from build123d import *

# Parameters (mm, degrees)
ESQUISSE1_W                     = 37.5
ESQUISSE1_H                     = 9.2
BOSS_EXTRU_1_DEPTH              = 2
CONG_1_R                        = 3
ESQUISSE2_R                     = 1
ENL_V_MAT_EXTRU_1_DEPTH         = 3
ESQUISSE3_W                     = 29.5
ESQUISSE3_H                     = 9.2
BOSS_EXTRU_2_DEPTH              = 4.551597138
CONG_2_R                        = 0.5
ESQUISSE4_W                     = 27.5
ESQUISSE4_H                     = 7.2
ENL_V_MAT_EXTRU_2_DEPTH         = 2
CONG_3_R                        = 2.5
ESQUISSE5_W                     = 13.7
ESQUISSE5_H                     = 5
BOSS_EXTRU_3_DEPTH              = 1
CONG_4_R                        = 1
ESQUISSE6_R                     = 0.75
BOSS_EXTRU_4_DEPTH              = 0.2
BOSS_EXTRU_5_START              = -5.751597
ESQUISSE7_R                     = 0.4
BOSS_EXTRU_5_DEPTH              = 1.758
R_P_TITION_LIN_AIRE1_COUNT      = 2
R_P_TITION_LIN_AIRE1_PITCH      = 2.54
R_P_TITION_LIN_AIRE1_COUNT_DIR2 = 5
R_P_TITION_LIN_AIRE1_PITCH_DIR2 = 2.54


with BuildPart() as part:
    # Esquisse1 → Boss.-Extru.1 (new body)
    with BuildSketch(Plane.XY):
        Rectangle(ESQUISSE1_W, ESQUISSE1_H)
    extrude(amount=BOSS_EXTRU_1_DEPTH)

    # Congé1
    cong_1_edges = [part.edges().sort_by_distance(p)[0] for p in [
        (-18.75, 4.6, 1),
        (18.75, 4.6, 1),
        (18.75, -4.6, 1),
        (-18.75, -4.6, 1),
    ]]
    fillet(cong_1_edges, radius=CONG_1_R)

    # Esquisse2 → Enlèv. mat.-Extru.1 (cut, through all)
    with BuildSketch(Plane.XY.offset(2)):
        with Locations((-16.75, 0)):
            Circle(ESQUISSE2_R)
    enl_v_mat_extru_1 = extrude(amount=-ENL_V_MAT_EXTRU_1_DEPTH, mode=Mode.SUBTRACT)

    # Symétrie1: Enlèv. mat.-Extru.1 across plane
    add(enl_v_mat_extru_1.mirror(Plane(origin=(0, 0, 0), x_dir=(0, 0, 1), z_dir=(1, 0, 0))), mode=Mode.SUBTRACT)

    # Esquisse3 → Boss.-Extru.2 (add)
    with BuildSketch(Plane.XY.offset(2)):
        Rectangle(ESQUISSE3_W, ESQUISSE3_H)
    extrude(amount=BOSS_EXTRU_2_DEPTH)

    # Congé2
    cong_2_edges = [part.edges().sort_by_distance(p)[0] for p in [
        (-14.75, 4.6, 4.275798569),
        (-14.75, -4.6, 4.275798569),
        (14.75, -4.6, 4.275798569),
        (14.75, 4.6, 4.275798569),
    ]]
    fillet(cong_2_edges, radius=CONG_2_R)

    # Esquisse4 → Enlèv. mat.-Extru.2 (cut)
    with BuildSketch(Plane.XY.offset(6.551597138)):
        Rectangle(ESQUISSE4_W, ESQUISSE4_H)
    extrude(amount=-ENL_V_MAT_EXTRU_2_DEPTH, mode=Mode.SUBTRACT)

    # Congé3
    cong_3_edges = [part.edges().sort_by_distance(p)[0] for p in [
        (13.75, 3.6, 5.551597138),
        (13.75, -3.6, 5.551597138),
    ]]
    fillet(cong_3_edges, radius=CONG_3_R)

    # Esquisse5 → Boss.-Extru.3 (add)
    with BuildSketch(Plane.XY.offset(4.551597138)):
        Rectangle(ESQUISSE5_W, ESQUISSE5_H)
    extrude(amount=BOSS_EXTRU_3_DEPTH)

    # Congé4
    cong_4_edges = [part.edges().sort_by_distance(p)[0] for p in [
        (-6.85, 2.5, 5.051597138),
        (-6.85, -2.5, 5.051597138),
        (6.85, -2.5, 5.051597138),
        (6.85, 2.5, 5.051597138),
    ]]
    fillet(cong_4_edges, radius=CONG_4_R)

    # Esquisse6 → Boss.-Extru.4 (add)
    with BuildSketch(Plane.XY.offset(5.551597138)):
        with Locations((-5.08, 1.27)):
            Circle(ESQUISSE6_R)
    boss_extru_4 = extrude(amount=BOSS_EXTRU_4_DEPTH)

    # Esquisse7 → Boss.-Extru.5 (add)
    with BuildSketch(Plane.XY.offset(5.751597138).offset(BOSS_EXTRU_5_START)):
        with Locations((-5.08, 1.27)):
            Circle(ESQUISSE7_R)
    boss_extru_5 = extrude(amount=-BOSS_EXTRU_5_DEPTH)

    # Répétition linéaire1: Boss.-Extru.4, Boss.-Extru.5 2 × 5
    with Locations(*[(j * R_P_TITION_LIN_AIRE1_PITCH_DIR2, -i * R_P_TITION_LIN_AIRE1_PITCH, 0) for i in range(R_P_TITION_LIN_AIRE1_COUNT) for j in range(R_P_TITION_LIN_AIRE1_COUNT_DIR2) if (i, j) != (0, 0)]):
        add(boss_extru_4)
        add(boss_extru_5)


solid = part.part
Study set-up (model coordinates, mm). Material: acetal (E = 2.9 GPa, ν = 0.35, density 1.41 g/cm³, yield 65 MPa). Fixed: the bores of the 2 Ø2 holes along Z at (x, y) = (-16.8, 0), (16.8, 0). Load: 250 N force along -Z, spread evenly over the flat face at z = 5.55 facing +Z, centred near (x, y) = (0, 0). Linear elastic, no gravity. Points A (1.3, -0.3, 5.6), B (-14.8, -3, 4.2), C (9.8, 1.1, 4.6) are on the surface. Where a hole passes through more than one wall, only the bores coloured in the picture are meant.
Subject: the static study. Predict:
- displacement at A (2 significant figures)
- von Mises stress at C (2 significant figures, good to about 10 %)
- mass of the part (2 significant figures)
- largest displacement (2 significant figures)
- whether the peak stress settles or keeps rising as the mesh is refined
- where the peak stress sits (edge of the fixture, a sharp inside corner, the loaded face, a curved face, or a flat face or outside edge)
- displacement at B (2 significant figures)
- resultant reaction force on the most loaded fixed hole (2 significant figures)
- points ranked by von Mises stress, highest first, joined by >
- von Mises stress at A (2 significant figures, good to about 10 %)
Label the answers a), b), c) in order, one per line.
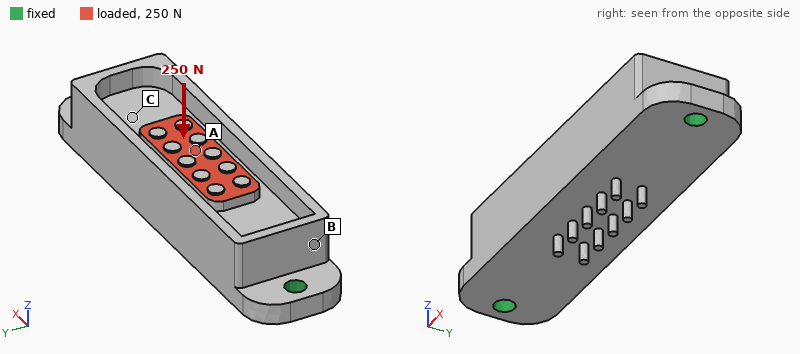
a) 0.27 mm
b) 11 MPa
c) 2.2 g
d) 0.28 mm
e) keeps rising
f) edge of the fixture
g) 0.066 mm
h) 220 N
i) A > C > B
j) 21 MPa
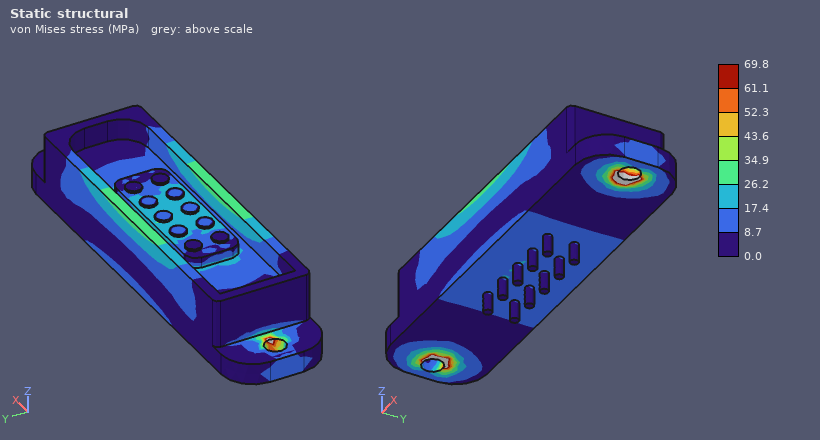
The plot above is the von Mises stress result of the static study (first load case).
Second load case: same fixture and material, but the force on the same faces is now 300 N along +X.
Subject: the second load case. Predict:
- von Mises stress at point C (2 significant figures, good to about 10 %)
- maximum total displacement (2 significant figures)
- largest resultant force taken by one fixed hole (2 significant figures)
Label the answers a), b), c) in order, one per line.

a) 5.0 MPa
b) 46 µm
c) 160 N
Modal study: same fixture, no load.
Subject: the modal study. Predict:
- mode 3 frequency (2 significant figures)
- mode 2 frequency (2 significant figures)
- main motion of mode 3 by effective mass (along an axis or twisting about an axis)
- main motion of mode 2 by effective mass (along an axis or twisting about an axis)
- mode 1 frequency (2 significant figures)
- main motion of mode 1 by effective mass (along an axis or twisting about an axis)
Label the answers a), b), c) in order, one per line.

a) 6300 Hz
b) 4200 Hz
c) along Y
d) along Z
e) 3800 Hz
f) along Y
